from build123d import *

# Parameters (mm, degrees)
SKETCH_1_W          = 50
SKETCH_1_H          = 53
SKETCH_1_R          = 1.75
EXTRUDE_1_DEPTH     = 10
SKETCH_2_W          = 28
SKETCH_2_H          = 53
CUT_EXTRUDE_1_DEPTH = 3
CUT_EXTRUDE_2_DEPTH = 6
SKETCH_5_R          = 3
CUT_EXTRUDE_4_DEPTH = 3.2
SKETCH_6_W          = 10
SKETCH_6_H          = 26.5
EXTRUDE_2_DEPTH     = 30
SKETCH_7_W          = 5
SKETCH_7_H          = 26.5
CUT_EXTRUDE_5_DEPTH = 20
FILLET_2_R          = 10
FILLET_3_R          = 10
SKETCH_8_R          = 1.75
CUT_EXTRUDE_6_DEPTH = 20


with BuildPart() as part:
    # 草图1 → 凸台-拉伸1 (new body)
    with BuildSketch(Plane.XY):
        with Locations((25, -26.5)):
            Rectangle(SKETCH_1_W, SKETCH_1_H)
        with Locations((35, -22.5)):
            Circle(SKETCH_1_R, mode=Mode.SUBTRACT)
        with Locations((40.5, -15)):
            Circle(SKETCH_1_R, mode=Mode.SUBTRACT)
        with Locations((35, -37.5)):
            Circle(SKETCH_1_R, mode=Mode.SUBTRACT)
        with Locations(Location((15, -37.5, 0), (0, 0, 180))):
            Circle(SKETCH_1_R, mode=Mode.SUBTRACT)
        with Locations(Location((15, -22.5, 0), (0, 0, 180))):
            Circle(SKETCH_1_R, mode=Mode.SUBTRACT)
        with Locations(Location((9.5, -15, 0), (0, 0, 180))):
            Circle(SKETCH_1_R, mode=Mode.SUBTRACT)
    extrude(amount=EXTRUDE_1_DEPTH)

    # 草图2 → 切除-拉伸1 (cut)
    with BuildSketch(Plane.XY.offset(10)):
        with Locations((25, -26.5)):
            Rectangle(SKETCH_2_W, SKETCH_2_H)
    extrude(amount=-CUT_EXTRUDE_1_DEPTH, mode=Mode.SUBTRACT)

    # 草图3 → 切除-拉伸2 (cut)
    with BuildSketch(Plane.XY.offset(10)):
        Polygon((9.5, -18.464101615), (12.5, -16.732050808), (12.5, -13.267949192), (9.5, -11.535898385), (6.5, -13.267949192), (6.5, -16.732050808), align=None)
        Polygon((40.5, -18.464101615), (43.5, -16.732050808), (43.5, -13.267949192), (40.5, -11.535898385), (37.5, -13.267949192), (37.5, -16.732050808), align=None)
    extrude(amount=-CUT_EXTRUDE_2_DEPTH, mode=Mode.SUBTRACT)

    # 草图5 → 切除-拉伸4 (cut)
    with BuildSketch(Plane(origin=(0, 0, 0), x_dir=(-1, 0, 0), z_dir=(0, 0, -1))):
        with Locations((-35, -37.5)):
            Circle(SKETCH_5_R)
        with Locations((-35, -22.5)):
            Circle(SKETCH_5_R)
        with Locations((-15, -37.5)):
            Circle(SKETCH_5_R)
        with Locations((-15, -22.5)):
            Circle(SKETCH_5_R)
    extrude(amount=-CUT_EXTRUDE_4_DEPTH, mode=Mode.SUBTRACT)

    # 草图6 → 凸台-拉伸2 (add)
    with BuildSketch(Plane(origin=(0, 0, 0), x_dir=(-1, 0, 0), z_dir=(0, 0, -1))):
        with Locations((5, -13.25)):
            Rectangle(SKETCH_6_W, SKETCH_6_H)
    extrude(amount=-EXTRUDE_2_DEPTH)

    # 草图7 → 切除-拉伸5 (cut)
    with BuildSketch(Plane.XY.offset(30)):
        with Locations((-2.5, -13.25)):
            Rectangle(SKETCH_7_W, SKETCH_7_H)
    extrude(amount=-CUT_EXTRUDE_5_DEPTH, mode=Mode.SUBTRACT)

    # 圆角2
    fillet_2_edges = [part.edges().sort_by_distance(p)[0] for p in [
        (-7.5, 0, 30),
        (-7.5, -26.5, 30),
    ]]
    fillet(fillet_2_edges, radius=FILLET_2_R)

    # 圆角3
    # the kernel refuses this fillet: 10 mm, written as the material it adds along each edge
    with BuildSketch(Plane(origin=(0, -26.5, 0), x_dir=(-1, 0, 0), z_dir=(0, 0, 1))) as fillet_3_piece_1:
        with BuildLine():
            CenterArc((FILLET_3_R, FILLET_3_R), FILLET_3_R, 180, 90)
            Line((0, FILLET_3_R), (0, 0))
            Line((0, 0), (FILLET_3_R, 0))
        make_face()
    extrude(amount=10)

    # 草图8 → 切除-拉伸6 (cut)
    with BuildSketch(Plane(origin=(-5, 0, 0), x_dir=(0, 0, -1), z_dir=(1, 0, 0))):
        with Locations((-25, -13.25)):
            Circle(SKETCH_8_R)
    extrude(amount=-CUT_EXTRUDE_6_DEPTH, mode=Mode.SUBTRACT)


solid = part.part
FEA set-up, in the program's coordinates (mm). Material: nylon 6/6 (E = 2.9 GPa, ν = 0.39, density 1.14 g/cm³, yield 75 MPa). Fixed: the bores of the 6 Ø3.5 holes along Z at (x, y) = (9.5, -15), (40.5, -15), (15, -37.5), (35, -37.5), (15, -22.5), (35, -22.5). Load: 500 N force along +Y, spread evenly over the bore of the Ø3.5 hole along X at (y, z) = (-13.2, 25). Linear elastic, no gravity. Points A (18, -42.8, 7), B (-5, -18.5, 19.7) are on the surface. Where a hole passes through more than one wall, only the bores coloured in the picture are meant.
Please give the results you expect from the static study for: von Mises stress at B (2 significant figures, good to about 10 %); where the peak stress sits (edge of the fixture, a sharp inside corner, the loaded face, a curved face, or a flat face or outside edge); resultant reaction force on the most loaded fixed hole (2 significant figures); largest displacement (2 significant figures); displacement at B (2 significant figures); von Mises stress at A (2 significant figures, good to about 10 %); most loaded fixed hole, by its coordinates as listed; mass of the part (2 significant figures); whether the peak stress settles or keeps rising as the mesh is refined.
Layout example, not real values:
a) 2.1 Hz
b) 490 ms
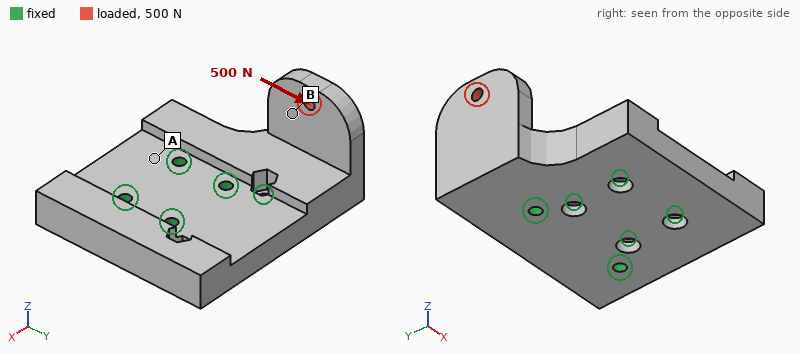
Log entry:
a) 11 MPa
b) edge of the fixture
c) 530 N
d) 0.88 mm
e) 0.54 mm
f) 4.5 MPa
g) (15, -37.5)
h) 30 g
i) keeps rising
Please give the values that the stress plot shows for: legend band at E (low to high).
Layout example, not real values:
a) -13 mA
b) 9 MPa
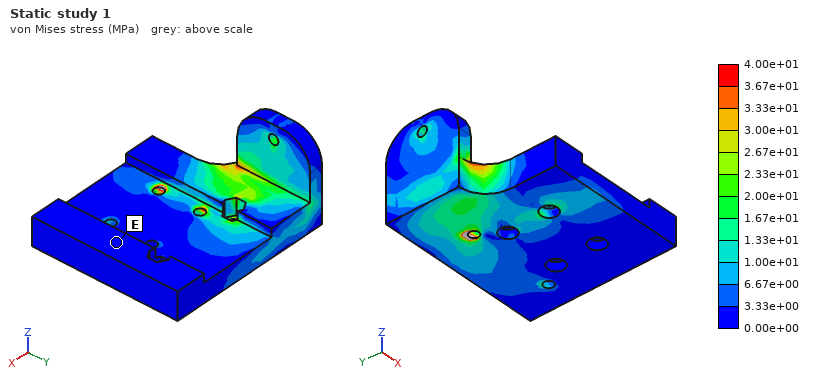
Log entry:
a) 0.00e+00 to 3.33e+00 MPa
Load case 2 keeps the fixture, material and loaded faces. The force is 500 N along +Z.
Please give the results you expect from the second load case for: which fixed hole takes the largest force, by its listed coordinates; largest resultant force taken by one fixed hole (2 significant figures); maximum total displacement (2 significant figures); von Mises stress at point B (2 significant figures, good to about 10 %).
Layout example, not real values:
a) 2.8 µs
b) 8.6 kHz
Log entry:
a) (9.5, -15)
b) 840 N
c) 0.87 mm
d) 5.3 MPa
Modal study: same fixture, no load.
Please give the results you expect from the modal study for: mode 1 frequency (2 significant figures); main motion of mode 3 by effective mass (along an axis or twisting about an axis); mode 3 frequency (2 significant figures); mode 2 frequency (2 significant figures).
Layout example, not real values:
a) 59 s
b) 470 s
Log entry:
a) 1700 Hz
b) along Z
c) 3500 Hz
d) 2600 Hz
